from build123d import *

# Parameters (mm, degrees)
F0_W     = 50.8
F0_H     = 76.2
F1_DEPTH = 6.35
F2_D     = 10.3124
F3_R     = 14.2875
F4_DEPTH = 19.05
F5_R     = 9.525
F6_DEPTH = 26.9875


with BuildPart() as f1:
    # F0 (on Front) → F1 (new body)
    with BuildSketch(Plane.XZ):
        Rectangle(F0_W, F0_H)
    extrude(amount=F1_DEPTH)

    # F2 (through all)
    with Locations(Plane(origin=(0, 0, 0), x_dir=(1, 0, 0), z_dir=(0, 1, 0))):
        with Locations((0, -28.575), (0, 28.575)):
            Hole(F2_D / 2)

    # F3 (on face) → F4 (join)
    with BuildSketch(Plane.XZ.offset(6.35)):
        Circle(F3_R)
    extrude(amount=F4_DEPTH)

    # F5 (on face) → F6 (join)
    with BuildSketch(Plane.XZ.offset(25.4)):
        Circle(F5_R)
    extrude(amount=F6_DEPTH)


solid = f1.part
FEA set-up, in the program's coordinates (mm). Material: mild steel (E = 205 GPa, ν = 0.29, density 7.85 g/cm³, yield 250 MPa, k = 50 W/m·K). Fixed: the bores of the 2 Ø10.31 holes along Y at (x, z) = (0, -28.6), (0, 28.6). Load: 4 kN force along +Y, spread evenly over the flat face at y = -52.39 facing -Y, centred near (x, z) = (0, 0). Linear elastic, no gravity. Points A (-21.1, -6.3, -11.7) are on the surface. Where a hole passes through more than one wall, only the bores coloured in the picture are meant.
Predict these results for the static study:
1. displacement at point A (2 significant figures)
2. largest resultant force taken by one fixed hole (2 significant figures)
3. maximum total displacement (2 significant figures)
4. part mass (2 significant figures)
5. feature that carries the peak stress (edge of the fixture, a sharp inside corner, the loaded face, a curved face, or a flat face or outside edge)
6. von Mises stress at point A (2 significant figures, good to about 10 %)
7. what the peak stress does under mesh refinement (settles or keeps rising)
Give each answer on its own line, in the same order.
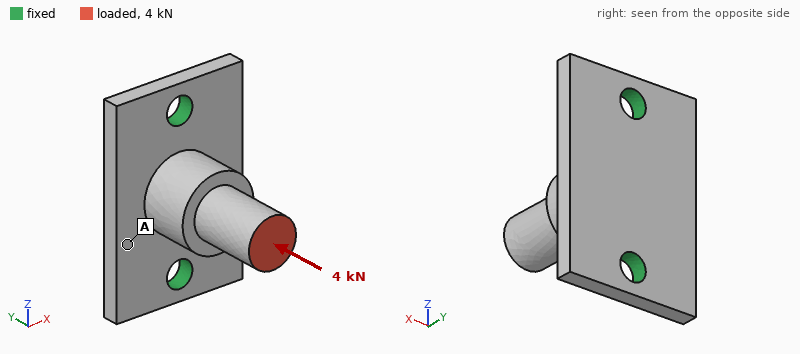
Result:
7.0 µm
2.1 kN
10 µm
340 g
edge of the fixture
11 MPa
keeps rising
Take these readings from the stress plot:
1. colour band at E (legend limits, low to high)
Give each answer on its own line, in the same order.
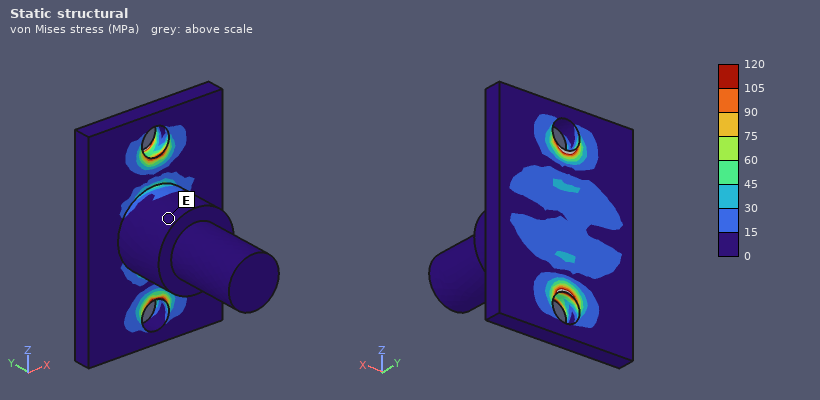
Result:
0 to 15 MPa
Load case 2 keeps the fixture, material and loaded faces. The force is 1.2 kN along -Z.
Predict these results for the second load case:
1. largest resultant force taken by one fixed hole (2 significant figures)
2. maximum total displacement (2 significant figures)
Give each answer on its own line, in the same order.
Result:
1.6 kN
29 µm
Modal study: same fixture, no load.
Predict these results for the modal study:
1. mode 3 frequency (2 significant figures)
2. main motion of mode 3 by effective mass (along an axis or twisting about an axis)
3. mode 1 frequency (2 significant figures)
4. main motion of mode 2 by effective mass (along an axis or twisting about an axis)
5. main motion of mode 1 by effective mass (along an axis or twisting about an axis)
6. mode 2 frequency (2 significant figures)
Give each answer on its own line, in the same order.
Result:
7100 Hz
along Y
2900 Hz
along Z
along X
5800 Hz
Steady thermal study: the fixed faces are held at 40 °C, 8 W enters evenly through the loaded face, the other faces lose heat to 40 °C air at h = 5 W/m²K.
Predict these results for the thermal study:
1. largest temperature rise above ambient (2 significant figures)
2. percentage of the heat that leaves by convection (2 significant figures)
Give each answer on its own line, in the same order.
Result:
27 K
4.5 %
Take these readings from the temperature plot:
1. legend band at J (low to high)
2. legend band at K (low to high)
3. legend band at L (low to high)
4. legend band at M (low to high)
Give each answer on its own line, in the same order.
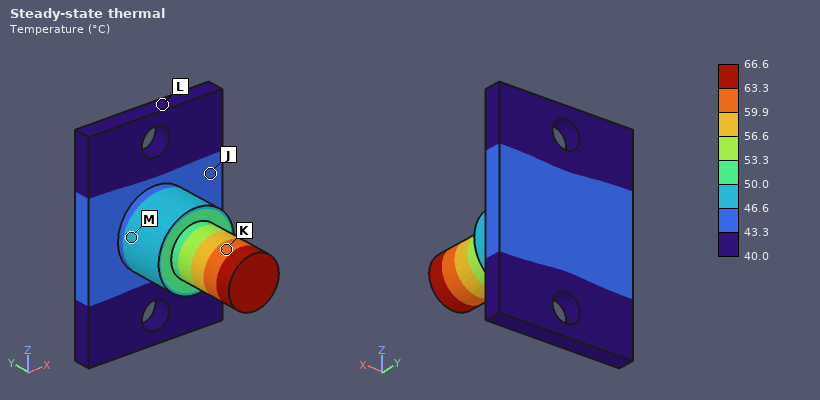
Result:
43.3 to 46.6 °C
59.9 to 63.3 °C
40.0 to 43.3 °C
46.6 to 50.0 °C
